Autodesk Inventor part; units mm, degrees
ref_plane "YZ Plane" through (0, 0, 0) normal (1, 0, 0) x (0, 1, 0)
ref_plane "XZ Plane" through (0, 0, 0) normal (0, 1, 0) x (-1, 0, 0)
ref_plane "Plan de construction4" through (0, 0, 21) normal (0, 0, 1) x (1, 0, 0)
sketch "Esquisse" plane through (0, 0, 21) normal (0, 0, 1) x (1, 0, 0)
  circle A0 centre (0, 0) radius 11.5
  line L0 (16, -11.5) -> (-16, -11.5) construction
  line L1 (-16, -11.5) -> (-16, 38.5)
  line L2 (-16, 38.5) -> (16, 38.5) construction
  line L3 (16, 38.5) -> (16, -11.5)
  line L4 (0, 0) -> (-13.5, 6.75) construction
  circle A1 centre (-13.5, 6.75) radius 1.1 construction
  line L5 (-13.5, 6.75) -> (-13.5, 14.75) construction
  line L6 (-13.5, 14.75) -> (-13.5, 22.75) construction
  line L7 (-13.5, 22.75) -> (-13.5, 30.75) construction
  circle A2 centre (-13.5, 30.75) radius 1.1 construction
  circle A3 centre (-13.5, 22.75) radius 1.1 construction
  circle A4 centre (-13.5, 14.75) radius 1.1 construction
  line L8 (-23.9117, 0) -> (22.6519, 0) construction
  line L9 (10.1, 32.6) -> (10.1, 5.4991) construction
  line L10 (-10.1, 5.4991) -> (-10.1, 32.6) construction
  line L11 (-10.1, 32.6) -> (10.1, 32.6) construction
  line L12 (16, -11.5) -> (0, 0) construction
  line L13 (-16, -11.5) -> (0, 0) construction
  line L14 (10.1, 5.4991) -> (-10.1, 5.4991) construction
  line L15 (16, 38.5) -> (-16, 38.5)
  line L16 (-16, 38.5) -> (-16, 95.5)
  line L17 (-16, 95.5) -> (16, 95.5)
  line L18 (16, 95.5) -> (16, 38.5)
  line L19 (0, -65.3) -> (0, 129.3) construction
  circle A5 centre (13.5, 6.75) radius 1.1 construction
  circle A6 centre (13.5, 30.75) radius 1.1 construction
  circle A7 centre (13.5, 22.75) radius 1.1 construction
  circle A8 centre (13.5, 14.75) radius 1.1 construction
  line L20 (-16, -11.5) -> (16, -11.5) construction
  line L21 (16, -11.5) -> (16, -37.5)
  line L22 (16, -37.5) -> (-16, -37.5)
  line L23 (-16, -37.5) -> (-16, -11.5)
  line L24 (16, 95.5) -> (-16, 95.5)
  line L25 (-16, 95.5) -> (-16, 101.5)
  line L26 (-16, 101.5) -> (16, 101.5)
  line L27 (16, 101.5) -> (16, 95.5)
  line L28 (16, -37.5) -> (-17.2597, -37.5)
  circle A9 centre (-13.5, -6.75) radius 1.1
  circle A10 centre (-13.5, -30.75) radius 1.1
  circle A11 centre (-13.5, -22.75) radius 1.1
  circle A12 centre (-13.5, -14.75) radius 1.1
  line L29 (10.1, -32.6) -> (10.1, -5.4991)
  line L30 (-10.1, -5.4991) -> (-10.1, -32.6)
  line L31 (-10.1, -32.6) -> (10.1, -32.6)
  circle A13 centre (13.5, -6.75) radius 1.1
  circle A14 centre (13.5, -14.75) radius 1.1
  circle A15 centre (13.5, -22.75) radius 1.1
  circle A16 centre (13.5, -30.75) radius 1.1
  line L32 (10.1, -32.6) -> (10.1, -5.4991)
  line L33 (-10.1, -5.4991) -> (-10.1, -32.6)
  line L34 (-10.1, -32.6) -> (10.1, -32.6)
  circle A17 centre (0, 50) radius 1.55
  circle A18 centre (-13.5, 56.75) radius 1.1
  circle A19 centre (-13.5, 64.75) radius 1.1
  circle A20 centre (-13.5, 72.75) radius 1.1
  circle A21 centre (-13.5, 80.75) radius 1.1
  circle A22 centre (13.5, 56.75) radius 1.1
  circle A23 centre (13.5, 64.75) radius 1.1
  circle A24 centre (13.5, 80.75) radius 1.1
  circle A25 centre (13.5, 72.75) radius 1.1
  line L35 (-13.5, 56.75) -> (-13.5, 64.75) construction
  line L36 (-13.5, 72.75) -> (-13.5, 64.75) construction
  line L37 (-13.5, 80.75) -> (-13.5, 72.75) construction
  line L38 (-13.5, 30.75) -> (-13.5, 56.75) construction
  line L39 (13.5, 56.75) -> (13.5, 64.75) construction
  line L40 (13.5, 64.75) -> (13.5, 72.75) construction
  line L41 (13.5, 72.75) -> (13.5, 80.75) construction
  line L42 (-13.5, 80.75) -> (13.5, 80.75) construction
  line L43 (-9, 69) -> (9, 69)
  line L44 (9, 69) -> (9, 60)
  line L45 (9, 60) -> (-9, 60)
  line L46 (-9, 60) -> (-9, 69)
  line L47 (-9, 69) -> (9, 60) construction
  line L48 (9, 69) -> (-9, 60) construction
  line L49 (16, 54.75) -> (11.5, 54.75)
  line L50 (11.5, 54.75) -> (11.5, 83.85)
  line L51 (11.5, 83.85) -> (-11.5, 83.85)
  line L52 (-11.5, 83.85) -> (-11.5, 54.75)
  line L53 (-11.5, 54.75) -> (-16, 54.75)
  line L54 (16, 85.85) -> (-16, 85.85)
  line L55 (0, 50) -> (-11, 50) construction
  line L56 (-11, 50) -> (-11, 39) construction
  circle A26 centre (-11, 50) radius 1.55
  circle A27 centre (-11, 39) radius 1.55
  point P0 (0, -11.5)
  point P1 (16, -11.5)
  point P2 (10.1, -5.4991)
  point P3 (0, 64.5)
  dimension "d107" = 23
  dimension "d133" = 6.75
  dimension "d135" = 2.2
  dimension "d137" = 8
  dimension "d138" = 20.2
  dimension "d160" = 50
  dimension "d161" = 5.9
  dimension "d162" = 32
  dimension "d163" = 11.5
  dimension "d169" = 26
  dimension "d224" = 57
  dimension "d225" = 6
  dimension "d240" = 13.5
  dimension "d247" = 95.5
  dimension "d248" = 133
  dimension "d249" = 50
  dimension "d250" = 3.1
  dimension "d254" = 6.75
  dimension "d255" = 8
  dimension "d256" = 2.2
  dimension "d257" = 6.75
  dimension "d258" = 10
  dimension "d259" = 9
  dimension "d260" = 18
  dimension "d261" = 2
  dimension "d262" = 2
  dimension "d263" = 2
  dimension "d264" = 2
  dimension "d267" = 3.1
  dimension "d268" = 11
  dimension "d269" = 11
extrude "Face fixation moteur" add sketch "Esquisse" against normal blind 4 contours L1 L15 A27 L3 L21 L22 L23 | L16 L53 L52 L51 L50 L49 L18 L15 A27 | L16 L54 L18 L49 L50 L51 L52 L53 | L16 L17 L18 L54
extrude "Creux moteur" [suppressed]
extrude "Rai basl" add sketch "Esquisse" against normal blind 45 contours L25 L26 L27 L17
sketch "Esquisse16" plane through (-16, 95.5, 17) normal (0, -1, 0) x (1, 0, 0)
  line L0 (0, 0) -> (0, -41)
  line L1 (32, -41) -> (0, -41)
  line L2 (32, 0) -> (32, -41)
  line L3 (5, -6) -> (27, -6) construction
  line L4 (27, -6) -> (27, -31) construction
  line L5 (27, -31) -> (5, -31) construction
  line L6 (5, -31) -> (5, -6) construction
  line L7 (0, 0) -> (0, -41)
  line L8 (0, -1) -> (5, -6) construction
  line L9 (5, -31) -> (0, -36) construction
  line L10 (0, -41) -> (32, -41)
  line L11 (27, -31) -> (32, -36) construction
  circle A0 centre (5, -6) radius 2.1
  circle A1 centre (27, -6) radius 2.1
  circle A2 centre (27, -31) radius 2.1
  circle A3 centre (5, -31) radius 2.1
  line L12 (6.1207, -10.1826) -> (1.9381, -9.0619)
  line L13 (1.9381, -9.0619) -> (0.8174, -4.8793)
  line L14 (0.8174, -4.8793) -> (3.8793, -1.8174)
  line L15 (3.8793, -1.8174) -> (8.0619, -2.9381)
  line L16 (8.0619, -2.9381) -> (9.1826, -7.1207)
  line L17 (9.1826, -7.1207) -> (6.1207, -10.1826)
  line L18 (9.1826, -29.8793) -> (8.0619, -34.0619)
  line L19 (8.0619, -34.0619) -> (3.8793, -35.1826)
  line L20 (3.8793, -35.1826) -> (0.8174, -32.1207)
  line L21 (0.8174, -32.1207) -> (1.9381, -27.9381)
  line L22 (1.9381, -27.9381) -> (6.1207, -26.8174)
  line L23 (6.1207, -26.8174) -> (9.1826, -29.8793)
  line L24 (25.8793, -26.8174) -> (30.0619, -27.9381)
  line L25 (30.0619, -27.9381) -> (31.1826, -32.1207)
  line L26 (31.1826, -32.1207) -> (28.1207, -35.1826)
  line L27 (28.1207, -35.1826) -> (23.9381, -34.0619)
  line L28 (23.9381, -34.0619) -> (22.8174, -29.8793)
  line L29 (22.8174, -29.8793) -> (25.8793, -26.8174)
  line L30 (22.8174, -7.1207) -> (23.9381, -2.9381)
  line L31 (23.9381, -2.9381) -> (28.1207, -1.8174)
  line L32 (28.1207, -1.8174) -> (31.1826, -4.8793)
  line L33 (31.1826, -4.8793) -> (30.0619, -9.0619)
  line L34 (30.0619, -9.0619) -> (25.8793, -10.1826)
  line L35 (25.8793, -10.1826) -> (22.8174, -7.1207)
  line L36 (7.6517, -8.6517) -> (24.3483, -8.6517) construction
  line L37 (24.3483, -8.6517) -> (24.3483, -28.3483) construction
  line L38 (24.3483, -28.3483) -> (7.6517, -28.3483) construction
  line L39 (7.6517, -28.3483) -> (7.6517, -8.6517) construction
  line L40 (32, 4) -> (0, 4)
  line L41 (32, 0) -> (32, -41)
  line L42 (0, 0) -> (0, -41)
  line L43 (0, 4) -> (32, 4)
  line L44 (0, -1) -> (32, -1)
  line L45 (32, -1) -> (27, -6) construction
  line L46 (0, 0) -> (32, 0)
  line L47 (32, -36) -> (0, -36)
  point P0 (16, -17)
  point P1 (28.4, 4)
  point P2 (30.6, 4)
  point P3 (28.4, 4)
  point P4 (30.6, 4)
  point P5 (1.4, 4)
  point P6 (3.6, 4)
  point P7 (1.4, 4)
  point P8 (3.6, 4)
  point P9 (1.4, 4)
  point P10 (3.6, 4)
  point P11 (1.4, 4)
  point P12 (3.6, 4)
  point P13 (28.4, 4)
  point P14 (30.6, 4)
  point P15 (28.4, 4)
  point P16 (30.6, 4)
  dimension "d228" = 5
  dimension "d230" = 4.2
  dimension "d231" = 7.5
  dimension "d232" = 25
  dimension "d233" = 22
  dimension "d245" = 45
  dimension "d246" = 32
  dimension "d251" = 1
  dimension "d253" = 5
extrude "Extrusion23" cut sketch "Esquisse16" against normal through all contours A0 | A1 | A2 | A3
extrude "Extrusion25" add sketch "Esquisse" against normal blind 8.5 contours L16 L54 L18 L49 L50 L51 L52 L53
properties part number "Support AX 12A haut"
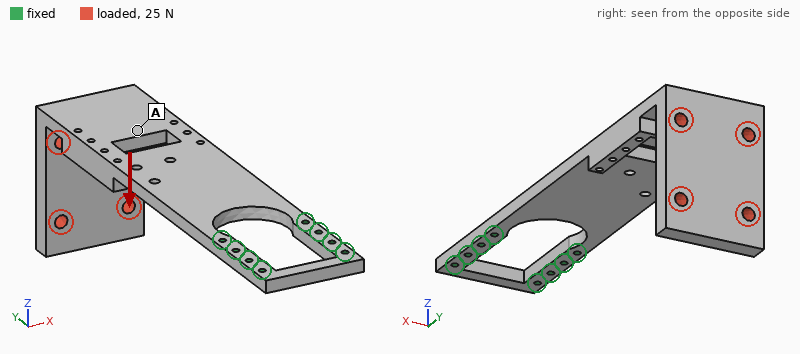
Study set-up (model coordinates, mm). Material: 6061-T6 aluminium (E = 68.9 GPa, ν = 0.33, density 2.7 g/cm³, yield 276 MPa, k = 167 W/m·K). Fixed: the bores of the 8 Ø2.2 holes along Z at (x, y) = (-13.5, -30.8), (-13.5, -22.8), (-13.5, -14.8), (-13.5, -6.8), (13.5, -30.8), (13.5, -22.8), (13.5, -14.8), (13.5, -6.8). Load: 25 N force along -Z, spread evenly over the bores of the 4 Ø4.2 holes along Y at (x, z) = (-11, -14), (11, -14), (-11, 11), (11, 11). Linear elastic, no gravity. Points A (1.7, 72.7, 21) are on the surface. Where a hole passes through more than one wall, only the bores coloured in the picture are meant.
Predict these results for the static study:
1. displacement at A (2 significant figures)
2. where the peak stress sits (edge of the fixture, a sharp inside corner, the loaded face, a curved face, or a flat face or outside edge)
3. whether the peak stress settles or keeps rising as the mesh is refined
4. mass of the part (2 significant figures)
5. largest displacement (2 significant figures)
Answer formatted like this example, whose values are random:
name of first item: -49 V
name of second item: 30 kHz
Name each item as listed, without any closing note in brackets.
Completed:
displacement at A: 1.1 mm
where the peak stress sits: edge of the fixture
whether the peak stress settles or keeps rising as the mesh is refined: keeps rising
mass of the part: 60 g
largest displacement: 1.8 mm
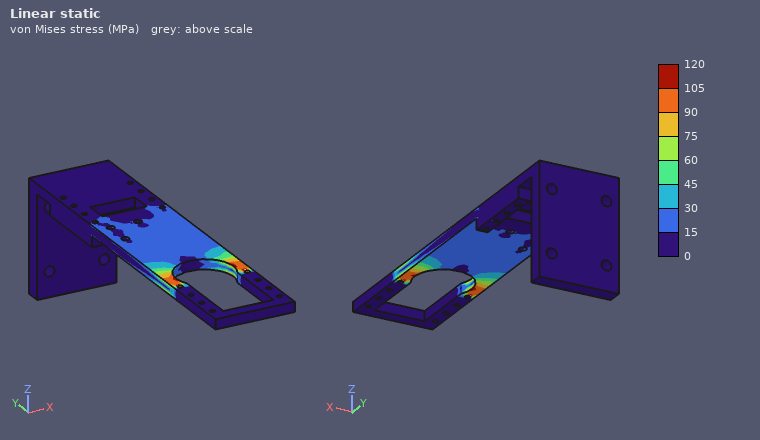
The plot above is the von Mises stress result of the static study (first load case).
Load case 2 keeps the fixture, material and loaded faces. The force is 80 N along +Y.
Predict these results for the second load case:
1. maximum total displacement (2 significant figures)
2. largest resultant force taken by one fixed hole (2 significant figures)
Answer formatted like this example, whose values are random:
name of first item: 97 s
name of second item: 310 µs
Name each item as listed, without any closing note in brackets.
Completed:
maximum total displacement: 1.5 mm
largest resultant force taken by one fixed hole: 40 N
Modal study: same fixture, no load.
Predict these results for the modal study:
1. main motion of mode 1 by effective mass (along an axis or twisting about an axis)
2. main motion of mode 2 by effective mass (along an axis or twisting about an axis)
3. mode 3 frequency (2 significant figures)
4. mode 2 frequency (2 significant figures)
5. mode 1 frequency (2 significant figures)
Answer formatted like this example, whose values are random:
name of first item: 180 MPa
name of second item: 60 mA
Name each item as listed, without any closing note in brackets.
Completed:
main motion of mode 1 by effective mass: along Z
main motion of mode 2 by effective mass: along X
mode 3 frequency: 810 Hz
mode 2 frequency: 470 Hz
mode 1 frequency: 110 Hz
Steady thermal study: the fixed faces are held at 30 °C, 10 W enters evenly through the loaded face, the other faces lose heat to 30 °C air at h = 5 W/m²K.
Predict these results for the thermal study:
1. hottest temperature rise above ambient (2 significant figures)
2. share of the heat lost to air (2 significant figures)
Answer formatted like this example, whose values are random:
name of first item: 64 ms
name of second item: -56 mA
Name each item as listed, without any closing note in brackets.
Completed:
hottest temperature rise above ambient: 63 K
share of the heat lost to air: 25 %
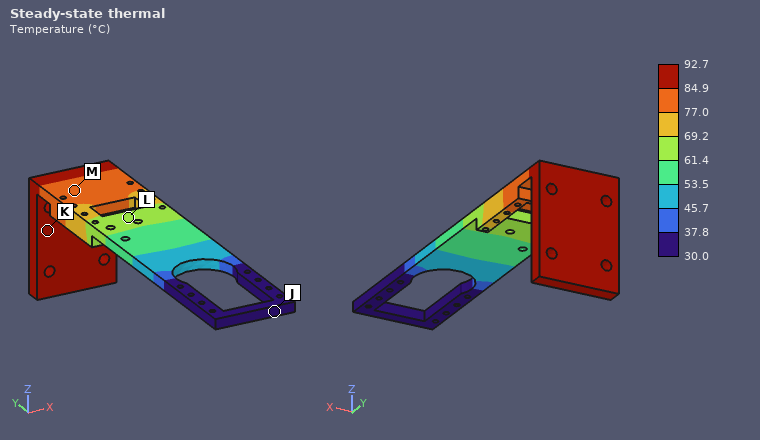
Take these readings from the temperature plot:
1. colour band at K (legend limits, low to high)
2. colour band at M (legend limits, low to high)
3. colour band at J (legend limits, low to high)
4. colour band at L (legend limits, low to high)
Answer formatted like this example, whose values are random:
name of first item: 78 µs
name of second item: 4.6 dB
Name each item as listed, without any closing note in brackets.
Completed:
colour band at K: 84.9 to 92.7 °C
colour band at M: 77.0 to 84.9 °C
colour band at J: 30.0 to 37.8 °C
colour band at L: 61.4 to 69.2 °C
